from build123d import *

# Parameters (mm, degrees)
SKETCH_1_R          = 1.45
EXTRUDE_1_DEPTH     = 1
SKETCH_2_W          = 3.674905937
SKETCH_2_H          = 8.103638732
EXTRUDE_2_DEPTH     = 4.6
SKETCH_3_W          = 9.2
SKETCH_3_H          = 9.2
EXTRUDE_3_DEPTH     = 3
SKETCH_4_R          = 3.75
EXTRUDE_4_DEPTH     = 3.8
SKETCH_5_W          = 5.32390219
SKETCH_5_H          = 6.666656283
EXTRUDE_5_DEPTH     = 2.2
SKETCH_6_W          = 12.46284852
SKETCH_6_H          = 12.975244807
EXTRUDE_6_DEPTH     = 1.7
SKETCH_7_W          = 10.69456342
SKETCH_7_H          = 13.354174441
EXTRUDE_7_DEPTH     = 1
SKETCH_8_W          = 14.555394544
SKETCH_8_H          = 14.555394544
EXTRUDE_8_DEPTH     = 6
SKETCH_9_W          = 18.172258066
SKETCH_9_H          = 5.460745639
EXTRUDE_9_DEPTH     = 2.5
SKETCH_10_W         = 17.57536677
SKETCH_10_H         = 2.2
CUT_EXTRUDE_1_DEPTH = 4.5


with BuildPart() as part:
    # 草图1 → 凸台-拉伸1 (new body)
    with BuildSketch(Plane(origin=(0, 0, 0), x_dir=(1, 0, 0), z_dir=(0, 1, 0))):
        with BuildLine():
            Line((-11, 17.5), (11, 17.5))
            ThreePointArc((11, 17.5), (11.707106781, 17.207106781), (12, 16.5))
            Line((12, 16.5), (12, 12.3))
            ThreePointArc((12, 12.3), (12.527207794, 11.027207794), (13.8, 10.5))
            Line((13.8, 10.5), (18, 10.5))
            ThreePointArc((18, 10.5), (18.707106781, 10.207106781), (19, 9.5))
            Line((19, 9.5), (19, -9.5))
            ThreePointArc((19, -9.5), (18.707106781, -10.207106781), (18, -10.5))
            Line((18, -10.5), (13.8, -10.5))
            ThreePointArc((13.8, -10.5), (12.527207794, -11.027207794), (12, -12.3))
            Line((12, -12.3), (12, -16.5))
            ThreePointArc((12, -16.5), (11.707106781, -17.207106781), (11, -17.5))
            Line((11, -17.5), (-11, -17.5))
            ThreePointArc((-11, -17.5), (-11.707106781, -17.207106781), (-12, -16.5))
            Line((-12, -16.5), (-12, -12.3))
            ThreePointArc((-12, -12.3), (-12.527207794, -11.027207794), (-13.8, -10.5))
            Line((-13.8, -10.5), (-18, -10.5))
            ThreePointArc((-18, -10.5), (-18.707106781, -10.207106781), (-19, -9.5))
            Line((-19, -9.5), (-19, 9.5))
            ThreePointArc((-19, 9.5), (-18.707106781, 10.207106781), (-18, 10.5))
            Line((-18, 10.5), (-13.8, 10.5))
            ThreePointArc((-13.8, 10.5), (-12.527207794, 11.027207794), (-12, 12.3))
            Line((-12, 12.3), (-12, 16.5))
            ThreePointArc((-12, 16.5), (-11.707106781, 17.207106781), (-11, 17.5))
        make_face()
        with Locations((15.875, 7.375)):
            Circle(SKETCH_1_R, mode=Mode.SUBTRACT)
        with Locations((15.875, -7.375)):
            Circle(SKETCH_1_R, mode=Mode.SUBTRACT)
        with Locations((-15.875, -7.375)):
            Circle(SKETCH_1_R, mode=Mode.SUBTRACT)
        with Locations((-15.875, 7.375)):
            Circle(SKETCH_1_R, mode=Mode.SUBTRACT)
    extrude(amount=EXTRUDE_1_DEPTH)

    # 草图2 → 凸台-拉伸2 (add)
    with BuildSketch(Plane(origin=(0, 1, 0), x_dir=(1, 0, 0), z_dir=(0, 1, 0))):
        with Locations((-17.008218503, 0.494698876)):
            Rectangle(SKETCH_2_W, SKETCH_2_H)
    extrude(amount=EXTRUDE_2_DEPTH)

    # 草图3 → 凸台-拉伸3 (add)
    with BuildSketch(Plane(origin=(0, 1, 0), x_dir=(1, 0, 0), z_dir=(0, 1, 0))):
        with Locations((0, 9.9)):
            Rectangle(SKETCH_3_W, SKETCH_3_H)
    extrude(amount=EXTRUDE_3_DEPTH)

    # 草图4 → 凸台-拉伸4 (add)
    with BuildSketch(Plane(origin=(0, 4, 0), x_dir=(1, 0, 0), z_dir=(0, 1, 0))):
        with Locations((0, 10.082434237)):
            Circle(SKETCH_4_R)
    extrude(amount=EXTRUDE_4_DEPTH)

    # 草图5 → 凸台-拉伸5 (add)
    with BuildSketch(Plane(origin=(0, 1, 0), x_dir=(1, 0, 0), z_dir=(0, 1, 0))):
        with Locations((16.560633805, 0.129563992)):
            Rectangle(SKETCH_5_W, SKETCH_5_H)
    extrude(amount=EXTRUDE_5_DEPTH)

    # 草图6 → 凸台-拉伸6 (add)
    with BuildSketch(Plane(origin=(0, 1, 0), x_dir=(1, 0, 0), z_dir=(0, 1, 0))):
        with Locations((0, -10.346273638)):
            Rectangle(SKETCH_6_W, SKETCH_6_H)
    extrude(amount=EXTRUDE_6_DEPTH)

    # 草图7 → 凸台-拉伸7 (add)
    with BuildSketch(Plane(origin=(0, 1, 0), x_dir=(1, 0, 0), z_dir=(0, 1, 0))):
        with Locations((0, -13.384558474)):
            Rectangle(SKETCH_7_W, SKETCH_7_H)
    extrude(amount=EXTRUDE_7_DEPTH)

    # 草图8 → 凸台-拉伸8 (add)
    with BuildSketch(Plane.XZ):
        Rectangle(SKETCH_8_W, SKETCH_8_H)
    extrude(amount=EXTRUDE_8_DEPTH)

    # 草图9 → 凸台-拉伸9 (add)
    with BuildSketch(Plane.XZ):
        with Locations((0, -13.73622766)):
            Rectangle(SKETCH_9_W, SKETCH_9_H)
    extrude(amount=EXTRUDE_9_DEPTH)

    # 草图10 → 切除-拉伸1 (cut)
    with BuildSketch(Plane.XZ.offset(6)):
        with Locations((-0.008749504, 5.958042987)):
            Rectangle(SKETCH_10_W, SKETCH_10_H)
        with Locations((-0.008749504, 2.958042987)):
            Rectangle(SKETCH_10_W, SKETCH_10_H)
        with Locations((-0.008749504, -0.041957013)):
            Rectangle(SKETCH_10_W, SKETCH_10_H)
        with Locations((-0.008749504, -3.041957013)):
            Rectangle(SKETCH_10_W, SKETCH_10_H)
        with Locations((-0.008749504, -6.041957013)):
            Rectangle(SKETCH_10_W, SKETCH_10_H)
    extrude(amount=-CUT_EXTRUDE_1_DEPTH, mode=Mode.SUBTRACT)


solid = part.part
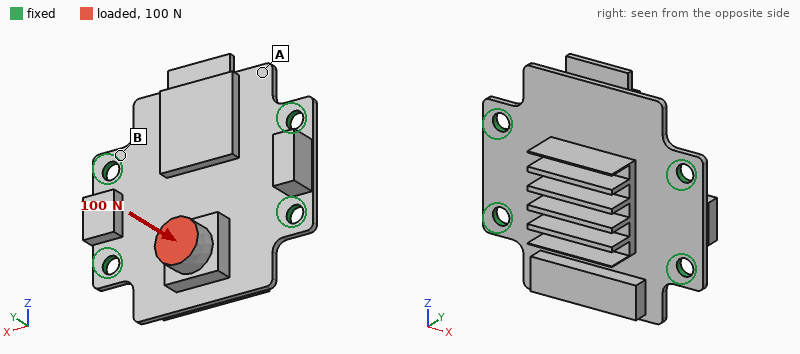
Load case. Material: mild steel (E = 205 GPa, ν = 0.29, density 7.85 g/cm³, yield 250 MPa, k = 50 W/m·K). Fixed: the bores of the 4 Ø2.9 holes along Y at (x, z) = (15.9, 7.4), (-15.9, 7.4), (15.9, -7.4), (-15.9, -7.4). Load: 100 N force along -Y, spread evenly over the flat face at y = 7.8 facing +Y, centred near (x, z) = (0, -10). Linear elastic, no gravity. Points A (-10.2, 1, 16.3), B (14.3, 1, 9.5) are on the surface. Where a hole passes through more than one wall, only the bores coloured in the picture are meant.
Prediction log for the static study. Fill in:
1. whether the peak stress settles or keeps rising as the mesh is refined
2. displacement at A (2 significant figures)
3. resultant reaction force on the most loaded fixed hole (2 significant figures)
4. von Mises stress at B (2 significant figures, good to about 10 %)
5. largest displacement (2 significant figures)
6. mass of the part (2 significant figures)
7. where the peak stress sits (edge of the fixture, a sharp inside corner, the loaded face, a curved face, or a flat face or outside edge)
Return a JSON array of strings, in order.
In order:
["keeps rising", "6.7 µm", "63 N", "20 MPa", "24 µm", "22 g", "edge of the fixture"]
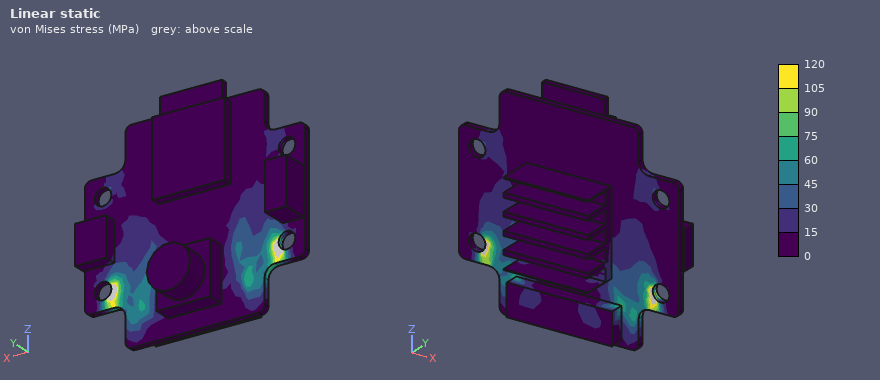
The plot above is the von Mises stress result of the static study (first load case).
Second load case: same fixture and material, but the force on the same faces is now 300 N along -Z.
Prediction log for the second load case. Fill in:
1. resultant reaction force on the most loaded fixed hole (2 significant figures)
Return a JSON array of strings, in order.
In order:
["120 N"]
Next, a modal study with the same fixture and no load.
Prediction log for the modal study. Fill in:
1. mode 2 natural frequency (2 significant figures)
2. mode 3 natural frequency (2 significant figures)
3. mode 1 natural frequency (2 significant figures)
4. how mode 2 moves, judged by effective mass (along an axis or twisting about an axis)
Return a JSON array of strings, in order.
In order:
["4700 Hz", "9400 Hz", "3700 Hz", "along Y"]
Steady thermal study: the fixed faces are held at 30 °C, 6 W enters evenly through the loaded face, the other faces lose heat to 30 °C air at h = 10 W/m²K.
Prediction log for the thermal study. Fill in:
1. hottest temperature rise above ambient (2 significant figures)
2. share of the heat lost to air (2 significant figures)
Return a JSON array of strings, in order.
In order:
["51 K", "12 %"]
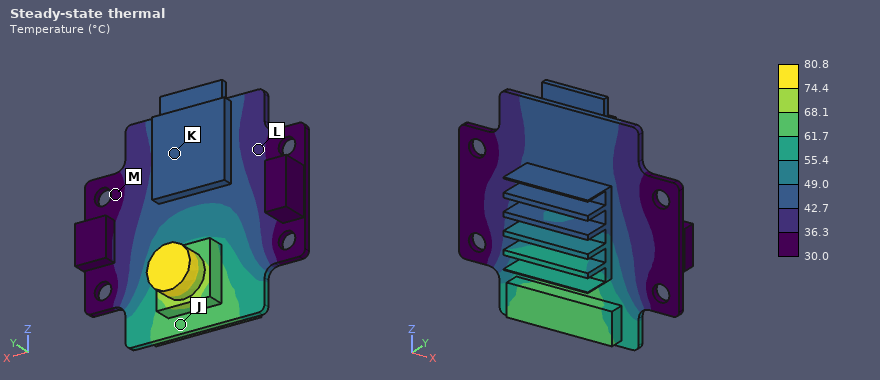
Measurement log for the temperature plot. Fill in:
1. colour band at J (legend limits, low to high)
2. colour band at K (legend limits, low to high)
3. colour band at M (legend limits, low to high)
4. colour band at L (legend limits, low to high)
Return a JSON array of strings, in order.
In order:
["61.7 to 68.1 °C", "42.7 to 49.0 °C", "30.0 to 36.3 °C", "36.3 to 42.7 °C"]
